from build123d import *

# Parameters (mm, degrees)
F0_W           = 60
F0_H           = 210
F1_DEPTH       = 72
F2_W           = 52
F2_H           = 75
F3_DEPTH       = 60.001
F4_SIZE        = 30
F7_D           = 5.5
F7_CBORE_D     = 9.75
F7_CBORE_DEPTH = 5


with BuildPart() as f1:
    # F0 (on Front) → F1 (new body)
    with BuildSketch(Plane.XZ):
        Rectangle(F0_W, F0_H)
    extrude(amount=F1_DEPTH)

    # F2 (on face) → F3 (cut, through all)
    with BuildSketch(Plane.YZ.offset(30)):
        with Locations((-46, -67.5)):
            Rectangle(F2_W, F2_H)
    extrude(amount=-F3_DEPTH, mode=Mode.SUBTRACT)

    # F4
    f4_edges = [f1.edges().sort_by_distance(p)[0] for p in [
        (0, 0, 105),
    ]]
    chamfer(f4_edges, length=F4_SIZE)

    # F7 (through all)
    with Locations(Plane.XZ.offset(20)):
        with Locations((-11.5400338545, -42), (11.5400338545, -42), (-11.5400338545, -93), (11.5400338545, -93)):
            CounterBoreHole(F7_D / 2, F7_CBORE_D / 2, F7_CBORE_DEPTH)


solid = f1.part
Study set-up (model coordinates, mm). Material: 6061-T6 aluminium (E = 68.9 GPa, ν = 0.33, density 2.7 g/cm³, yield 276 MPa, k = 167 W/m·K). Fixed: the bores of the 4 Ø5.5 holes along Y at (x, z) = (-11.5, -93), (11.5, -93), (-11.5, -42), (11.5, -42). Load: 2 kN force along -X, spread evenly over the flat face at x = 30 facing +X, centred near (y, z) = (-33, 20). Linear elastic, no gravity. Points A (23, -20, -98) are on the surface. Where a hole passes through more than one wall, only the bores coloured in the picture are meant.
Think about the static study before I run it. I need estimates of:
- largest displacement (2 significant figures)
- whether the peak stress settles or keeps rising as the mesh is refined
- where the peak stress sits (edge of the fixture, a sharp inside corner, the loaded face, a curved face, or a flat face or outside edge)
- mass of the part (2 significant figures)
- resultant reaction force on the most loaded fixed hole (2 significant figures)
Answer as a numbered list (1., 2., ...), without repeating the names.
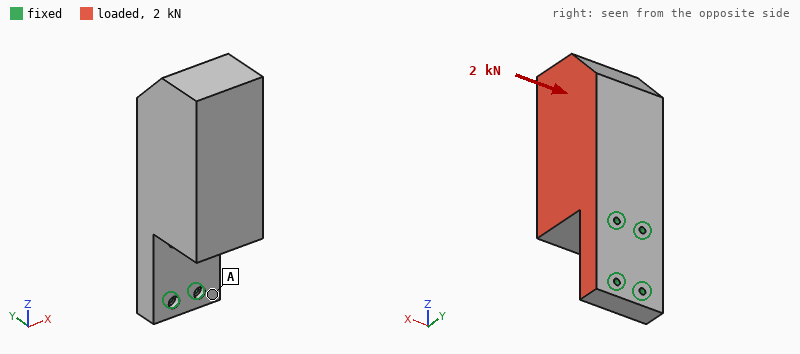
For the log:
1. 47 µm
2. keeps rising
3. edge of the fixture
4. 1.7 kg
5. 3.5 kN
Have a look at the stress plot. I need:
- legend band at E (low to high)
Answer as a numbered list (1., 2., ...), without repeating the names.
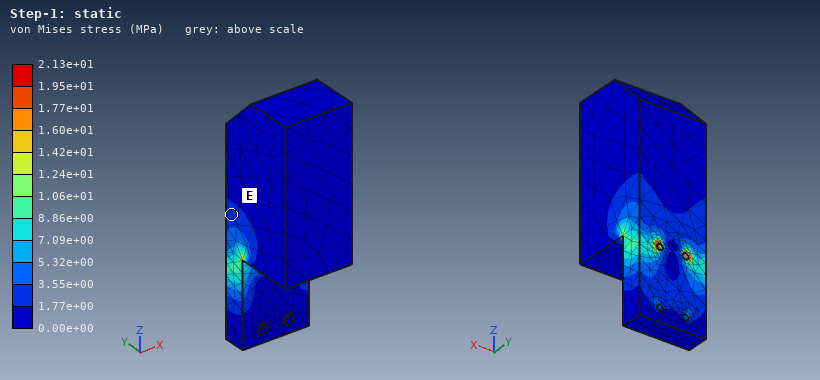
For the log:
1. 1.77e+00 to 3.55e+00 MPa
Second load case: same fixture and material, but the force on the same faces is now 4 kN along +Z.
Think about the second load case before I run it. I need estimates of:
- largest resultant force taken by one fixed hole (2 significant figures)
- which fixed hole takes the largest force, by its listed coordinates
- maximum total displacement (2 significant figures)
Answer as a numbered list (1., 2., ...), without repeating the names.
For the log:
1. 3.6 kN
2. (11.5, -42)
3. 0.17 mm
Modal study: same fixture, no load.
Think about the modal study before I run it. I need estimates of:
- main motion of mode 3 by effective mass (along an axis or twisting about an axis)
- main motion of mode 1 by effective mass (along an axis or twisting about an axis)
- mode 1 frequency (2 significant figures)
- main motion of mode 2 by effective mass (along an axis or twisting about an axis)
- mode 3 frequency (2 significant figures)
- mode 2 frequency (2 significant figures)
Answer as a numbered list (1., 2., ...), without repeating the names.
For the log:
1. twisting about Z
2. along Y
3. 450 Hz
4. along X
5. 2000 Hz
6. 1000 Hz
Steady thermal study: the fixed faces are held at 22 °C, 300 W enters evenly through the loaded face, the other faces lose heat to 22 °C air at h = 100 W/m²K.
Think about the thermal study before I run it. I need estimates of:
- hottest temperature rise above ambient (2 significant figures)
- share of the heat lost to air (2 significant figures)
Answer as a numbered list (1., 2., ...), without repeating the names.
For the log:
1. 40 K
2. 35 %
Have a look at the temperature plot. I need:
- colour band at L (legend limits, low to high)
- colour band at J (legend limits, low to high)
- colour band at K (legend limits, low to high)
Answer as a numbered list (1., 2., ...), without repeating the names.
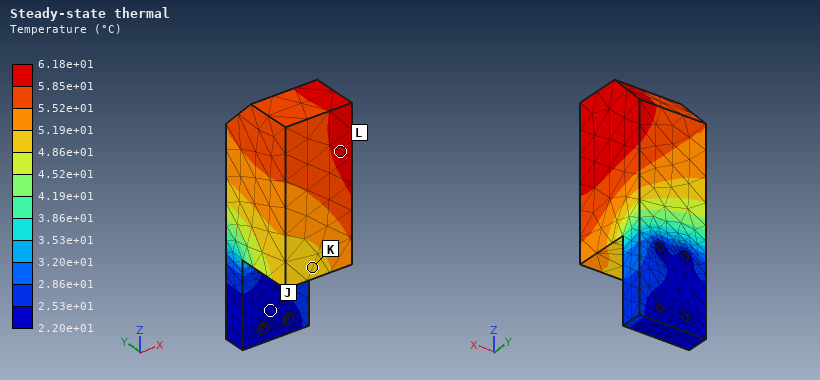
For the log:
1. 5.85e+01 to 6.18e+01 °C
2. 2.20e+01 to 2.53e+01 °C
3. 4.86e+01 to 5.19e+01 °C
